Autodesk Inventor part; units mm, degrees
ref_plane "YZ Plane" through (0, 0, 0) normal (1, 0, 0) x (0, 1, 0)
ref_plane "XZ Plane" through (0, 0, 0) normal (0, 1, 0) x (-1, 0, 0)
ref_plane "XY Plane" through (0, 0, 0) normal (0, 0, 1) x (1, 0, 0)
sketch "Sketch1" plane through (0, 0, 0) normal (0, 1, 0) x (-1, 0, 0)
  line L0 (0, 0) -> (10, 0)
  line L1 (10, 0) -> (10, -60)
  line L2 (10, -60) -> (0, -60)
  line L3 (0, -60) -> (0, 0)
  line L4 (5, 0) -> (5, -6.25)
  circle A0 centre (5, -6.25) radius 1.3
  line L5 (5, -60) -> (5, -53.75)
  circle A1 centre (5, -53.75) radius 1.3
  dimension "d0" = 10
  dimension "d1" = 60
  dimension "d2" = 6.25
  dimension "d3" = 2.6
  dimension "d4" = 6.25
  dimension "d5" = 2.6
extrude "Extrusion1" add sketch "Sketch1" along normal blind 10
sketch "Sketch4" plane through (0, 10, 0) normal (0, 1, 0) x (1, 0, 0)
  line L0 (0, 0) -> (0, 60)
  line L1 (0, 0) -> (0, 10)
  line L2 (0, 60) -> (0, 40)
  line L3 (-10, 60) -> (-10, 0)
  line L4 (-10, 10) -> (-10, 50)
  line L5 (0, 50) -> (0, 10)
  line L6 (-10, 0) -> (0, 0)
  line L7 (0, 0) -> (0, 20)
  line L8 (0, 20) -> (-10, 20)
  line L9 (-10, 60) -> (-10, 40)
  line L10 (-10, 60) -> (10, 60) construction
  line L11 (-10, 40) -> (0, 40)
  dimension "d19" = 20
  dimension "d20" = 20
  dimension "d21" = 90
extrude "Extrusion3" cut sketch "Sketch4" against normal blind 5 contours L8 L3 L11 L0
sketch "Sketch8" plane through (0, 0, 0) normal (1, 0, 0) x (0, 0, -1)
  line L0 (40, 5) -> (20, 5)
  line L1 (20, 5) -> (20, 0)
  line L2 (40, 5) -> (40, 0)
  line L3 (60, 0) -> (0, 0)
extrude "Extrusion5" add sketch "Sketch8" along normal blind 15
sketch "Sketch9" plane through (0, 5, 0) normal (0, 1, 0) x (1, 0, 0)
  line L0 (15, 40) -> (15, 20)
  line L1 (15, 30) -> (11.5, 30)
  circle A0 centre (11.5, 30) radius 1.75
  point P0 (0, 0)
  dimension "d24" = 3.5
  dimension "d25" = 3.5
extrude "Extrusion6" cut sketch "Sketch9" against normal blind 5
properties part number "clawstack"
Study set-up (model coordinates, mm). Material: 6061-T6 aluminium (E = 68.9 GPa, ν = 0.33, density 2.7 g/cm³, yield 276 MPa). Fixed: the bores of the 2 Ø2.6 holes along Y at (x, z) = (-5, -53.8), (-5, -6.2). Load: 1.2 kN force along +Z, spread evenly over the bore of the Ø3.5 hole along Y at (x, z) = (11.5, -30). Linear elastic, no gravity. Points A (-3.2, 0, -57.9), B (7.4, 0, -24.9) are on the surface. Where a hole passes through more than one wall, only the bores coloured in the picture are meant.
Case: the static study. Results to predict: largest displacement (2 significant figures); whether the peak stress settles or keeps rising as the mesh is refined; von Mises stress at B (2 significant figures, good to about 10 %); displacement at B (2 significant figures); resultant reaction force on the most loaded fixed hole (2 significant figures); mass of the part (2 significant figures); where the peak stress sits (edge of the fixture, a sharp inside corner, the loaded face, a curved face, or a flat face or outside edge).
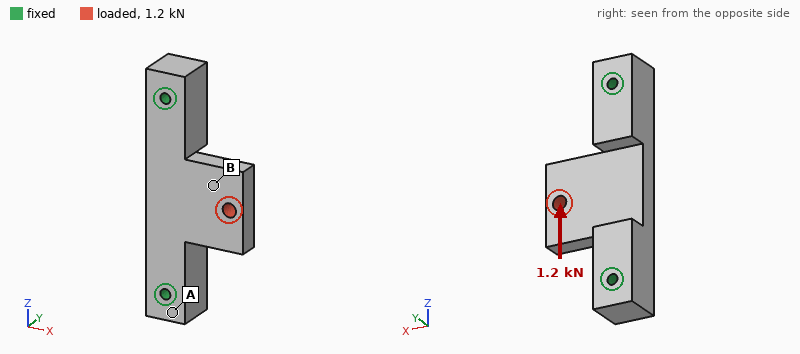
34 µm
keeps rising
21 MPa
18 µm
790 N
17 g
a sharp inside corner
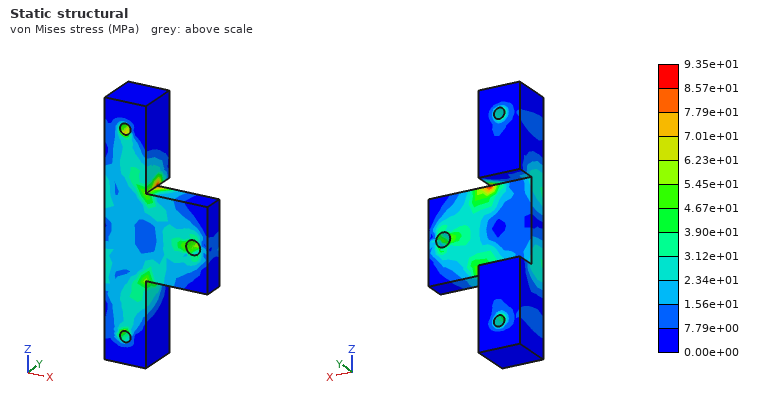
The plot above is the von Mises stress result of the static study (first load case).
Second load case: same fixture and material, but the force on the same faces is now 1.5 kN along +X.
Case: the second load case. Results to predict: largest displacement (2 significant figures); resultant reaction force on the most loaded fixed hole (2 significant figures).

39 µm
800 N
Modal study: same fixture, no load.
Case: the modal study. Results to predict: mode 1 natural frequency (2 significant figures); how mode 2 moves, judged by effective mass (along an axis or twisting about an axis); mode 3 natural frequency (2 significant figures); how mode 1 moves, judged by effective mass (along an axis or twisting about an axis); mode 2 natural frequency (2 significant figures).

7400 Hz
along X
19 kHz
along Y
13 kHz
